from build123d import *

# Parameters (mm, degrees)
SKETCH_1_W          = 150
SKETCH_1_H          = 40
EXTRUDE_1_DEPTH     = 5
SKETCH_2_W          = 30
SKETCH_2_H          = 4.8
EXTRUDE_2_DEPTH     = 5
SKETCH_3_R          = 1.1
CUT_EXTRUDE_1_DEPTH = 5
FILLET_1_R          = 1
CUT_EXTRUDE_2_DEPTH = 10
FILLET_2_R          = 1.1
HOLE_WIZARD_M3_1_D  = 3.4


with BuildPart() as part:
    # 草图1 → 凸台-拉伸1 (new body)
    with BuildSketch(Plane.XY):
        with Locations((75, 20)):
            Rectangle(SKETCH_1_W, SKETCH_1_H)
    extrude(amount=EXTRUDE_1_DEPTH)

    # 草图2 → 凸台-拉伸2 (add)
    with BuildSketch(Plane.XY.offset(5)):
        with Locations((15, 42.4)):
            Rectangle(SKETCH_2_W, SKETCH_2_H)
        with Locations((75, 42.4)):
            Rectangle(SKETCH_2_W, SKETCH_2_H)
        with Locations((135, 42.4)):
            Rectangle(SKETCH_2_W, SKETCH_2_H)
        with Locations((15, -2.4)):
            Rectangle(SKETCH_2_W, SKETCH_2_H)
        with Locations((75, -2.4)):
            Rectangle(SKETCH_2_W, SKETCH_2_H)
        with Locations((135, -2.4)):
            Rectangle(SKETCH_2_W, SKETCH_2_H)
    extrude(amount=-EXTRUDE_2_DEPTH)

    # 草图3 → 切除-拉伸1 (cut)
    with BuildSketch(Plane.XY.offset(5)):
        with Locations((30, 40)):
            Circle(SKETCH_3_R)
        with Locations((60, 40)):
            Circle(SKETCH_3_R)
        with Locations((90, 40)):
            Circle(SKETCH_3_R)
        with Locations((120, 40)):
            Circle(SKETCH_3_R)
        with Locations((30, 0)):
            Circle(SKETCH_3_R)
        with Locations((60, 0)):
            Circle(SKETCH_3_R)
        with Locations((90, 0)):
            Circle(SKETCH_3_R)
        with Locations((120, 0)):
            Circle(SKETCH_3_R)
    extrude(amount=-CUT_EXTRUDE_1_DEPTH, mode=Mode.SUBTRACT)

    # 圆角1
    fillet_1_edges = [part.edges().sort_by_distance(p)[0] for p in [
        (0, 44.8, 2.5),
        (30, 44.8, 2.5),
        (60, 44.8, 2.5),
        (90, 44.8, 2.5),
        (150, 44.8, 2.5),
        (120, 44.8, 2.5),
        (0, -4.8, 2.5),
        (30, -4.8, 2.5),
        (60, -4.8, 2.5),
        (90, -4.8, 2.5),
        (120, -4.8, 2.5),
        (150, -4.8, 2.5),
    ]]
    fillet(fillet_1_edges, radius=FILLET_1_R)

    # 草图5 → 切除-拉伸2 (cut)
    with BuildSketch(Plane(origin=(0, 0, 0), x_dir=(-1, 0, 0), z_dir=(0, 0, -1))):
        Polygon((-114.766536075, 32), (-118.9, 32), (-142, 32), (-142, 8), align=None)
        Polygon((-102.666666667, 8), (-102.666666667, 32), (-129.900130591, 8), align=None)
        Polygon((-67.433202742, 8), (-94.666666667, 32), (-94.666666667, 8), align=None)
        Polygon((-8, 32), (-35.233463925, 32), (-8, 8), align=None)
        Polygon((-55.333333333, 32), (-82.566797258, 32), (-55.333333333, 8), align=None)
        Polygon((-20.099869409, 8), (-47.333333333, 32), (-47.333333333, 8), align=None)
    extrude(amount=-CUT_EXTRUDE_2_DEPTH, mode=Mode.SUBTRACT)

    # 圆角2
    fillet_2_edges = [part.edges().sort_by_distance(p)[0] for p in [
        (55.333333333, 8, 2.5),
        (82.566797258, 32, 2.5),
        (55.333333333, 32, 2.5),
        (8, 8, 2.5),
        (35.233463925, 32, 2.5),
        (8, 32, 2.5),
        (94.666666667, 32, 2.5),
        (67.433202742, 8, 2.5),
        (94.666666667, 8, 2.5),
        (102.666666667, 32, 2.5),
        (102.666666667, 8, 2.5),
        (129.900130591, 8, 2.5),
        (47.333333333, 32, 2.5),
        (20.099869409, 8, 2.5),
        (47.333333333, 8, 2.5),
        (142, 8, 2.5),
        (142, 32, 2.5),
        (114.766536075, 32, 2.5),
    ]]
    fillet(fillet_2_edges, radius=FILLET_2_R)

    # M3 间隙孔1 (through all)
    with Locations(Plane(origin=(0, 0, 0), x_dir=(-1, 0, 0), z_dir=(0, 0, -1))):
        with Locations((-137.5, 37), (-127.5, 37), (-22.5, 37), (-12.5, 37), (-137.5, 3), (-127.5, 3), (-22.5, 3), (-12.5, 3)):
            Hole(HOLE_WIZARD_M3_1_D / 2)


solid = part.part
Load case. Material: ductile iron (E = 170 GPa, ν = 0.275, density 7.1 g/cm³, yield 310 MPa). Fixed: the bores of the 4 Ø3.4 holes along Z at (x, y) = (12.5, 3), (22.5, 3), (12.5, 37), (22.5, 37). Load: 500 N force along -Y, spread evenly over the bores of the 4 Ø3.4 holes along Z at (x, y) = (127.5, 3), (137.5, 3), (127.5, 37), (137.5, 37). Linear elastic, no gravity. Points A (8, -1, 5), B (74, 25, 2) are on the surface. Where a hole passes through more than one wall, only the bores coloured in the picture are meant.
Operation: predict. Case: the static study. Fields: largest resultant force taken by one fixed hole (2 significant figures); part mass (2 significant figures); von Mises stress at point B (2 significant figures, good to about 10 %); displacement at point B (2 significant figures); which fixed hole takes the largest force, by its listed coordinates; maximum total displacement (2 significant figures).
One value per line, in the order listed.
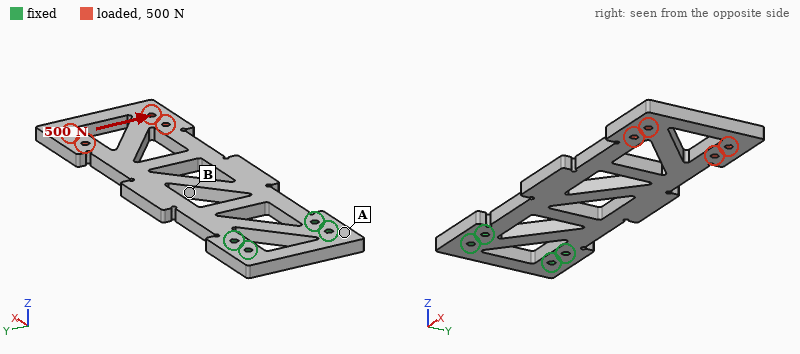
1.5 kN
170 g
20 MPa
0.033 mm
(22.5, 37)
0.11 mm
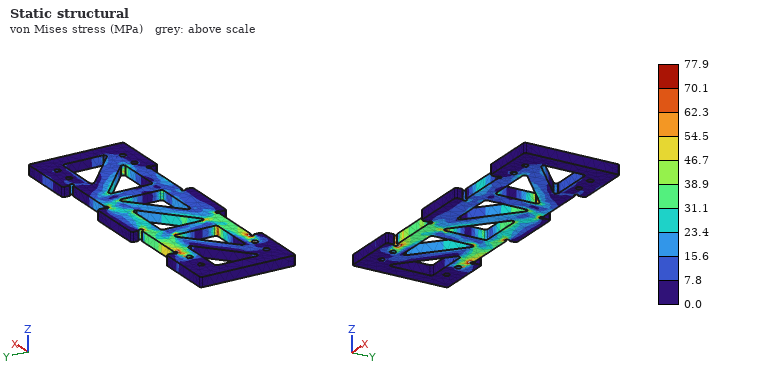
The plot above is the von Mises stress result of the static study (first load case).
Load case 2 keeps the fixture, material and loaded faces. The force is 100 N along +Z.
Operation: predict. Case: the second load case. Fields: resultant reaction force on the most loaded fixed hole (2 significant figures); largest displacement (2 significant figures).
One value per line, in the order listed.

260 N
1.5 mm
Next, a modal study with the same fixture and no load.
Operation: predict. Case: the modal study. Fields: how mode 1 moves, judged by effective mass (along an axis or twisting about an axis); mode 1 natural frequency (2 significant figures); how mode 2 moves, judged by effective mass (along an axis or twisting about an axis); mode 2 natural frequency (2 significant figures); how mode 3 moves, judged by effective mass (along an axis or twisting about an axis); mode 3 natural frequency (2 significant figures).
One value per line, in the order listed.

along Z
190 Hz
twisting about X
960 Hz
along Z
1200 Hz
